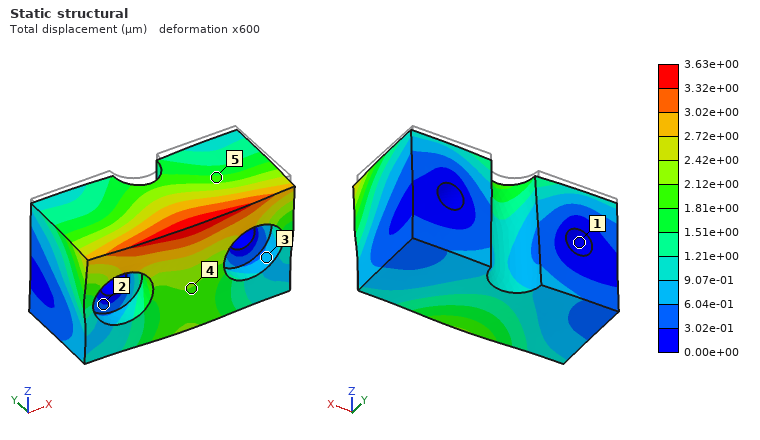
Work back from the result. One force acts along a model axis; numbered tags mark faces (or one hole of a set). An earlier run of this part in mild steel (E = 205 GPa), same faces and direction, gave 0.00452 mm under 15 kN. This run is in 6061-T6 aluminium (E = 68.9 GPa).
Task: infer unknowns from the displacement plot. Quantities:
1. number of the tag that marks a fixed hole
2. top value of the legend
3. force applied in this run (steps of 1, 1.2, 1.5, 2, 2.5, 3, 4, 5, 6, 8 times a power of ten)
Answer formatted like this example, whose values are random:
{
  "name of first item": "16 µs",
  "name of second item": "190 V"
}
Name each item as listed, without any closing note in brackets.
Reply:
{
  "number of the tag that marks a fixed hole": "1",
  "top value of the legend": "3.63e+00 µm",
  "force applied in this run": "4 kN"
}
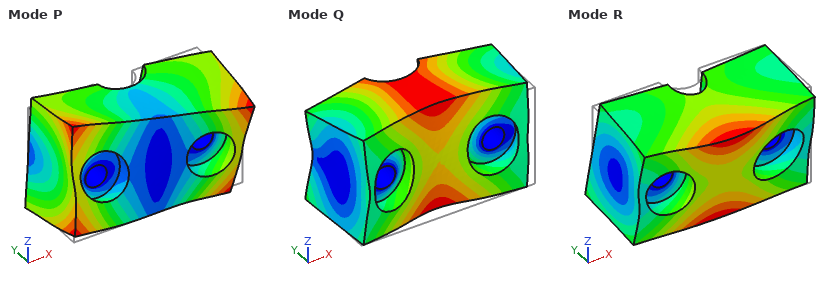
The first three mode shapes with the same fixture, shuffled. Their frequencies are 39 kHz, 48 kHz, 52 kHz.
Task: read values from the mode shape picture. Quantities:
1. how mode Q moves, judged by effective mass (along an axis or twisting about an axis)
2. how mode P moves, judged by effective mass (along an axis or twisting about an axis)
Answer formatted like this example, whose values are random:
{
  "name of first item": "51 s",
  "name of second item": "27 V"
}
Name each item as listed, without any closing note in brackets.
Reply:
{
  "how mode Q moves, judged by effective mass": "along Y",
  "how mode P moves, judged by effective mass": "twisting about Y"
}
